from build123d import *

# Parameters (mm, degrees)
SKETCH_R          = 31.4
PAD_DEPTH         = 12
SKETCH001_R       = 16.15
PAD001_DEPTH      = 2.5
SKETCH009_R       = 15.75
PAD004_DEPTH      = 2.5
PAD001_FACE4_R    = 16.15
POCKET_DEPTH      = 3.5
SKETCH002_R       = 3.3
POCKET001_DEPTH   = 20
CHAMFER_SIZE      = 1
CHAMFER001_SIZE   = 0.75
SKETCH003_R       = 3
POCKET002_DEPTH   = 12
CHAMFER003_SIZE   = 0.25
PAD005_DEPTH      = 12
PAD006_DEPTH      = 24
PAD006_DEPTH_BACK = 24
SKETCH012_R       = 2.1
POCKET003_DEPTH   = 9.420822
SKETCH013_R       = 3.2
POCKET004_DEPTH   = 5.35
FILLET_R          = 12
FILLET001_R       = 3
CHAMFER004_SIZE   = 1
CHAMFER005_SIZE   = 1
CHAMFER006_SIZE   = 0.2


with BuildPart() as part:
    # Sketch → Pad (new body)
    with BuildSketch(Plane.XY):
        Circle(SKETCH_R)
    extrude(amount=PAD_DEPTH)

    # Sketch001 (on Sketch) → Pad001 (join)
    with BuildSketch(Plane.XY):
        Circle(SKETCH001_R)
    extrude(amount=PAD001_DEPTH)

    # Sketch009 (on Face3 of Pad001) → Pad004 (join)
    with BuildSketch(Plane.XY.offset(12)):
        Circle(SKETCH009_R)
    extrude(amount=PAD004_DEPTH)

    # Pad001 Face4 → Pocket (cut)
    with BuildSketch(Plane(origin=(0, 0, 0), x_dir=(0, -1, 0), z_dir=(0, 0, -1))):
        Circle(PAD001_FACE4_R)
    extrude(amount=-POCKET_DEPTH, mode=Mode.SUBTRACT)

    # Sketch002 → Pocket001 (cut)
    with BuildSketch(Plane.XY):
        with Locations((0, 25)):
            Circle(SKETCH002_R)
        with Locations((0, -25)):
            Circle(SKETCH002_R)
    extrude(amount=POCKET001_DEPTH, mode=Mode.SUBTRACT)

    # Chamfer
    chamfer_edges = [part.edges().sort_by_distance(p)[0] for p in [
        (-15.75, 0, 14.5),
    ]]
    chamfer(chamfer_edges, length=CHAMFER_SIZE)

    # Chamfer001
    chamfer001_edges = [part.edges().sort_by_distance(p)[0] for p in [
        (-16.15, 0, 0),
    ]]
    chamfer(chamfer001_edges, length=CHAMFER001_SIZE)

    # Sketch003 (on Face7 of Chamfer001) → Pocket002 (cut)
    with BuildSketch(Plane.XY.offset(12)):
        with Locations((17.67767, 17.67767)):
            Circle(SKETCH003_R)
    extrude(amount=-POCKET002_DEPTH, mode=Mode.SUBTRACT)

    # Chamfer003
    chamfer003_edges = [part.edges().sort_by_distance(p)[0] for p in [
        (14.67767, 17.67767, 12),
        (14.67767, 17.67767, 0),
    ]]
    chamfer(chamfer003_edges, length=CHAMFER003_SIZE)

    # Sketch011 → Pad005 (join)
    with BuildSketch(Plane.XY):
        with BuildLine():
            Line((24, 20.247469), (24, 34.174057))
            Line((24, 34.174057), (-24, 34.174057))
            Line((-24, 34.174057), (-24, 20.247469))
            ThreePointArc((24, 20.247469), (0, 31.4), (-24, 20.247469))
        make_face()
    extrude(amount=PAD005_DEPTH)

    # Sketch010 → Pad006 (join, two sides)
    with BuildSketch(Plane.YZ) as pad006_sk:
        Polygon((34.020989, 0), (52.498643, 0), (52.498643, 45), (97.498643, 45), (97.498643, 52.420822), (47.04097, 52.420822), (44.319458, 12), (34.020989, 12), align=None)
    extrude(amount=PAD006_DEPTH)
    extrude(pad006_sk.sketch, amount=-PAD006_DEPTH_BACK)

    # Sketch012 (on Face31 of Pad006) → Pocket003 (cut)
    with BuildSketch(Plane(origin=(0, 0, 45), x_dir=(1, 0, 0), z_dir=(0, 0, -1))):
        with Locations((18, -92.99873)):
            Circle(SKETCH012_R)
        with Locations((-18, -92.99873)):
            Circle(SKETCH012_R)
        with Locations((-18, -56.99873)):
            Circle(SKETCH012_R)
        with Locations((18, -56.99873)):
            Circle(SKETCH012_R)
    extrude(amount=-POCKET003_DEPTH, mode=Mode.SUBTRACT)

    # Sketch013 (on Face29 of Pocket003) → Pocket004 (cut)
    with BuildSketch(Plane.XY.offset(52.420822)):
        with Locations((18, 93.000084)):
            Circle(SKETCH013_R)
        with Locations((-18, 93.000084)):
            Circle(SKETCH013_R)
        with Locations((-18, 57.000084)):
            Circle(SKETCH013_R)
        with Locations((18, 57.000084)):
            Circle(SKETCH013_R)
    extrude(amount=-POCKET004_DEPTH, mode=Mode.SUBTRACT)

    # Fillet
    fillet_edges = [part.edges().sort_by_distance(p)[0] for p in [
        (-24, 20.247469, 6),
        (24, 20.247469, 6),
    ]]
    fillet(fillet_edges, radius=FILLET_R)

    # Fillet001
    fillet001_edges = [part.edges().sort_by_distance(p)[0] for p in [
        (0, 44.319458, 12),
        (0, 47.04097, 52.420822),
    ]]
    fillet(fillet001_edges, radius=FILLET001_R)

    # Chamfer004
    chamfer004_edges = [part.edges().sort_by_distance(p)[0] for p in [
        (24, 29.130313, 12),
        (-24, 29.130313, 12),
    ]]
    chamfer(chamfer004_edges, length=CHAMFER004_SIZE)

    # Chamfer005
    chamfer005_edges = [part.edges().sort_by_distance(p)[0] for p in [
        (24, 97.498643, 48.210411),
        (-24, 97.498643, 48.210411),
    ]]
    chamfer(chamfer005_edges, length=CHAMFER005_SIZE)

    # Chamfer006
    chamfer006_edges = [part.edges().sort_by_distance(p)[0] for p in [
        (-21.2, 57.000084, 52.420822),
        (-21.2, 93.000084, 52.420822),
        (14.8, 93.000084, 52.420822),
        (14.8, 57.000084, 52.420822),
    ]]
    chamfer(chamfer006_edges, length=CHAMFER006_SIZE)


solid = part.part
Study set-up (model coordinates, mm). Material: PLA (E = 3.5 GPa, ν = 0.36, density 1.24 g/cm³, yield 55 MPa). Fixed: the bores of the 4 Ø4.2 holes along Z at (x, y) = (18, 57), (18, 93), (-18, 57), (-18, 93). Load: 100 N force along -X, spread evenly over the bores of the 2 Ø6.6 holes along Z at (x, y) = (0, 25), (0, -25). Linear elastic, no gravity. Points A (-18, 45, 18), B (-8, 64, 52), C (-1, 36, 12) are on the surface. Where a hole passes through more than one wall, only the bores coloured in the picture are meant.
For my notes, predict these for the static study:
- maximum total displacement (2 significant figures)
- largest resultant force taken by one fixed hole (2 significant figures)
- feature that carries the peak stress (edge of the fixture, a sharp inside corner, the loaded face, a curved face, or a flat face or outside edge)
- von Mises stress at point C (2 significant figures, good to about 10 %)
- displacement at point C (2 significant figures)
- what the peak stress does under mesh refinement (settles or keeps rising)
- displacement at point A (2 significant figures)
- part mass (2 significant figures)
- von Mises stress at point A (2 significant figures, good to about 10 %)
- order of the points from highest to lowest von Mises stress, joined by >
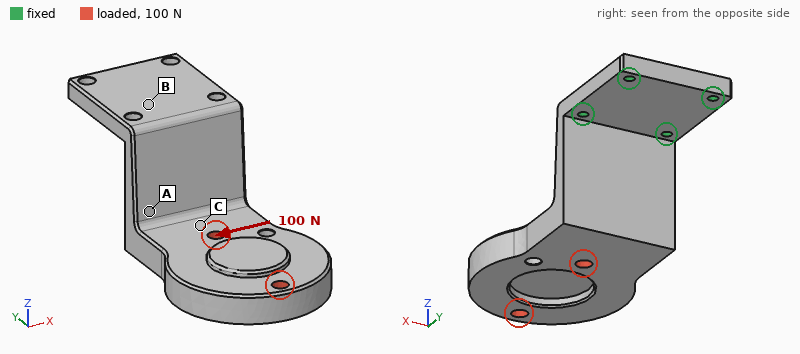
1.3 mm
180 N
edge of the fixture
2.1 MPa
0.22 mm
keeps rising
0.25 mm
96 g
7.9 MPa
A > C > B
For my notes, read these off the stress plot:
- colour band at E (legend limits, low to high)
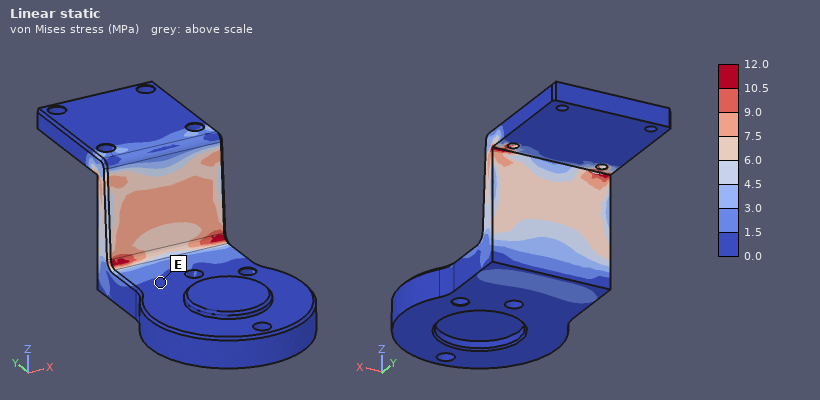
0.0 to 1.5 MPa
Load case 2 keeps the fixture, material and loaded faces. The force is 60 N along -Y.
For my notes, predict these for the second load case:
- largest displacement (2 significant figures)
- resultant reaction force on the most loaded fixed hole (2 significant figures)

1.7 mm
97 N
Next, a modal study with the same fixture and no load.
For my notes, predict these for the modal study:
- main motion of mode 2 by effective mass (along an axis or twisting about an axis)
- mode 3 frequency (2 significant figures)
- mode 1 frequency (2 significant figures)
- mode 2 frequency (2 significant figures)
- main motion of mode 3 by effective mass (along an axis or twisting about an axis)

along X
560 Hz
110 Hz
240 Hz
along Y
